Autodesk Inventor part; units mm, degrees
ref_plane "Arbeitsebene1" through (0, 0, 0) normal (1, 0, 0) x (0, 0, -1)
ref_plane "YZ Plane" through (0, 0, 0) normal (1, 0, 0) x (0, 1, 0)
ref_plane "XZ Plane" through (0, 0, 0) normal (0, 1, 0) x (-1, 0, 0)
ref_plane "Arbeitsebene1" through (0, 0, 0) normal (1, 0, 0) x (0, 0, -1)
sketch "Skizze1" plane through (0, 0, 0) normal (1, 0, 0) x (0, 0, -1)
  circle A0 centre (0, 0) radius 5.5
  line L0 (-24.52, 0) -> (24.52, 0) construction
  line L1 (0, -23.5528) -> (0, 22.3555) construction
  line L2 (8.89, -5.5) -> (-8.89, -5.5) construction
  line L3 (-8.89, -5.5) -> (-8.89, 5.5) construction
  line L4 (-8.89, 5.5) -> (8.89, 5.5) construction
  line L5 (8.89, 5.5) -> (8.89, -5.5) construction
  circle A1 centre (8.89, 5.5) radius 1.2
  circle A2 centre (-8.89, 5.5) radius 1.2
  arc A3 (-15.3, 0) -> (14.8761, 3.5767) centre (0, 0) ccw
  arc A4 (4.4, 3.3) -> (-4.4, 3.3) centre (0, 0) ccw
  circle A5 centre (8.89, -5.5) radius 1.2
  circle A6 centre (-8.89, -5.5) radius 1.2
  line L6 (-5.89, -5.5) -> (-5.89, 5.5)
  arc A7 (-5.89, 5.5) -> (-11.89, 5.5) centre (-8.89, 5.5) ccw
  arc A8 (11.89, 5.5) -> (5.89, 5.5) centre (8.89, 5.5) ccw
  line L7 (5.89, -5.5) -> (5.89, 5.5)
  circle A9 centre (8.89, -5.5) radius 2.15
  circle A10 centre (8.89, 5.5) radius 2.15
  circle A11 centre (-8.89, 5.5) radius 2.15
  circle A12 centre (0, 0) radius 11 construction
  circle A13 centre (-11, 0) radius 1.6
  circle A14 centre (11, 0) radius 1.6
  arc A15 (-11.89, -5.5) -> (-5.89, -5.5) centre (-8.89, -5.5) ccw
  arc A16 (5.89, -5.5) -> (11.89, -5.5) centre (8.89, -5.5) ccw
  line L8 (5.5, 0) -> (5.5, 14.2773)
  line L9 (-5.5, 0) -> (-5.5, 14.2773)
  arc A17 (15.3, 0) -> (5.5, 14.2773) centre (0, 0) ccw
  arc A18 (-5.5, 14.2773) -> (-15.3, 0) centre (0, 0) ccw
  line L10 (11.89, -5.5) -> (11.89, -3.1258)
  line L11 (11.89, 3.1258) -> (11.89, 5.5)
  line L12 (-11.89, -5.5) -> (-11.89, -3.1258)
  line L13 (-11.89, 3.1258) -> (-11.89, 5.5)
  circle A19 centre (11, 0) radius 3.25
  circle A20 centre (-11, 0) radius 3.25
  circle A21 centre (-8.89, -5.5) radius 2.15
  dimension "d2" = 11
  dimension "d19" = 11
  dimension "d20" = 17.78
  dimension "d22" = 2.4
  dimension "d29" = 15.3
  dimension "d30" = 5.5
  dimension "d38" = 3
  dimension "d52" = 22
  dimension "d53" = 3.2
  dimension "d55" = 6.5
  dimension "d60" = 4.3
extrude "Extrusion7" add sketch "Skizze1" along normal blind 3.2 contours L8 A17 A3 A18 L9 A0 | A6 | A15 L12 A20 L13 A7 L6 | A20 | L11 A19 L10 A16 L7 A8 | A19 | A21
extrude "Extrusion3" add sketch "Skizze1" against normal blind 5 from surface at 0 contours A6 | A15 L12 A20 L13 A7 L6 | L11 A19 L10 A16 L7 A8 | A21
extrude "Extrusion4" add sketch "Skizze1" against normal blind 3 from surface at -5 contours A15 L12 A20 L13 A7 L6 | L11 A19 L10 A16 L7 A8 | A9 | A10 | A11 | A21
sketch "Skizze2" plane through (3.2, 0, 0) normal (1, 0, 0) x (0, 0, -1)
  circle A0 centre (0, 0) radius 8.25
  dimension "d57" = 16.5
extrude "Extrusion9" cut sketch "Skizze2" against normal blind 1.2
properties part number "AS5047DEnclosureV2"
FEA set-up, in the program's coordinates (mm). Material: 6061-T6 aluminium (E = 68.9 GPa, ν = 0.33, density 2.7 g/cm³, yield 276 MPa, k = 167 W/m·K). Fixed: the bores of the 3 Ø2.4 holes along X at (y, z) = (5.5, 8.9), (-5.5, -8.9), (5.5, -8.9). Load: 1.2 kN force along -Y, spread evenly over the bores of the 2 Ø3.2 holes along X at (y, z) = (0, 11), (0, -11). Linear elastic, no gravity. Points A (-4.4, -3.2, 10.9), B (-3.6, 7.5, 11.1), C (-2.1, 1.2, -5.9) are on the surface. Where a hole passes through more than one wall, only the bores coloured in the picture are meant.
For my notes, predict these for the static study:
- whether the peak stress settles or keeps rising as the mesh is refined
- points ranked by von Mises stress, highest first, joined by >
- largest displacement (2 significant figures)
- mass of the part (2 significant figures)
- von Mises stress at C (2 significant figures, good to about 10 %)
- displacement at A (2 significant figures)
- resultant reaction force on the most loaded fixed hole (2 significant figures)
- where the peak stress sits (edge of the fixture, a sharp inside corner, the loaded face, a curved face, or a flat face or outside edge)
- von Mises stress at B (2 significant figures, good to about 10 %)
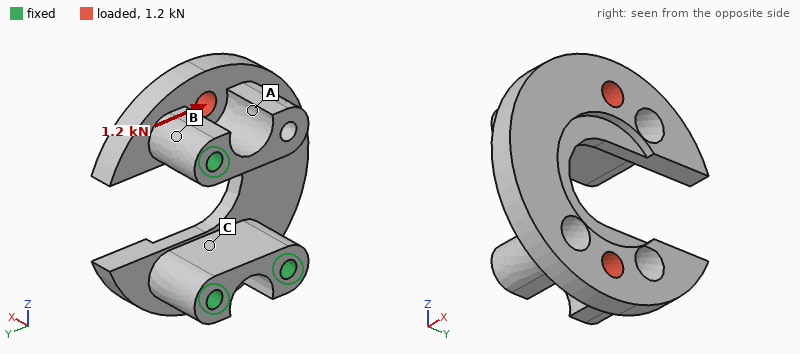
keeps rising
B > C > A
83 µm
6.1 g
38 MPa
43 µm
590 N
edge of the fixture
100 MPa
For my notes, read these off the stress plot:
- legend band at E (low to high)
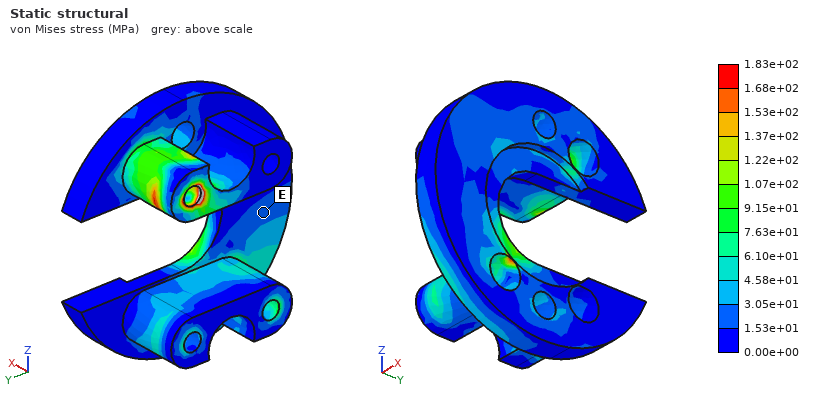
1.53e+01 to 3.05e+01 MPa
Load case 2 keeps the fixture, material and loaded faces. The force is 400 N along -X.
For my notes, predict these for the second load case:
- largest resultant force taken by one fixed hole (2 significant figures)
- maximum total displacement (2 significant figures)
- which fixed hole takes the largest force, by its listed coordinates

190 N
23 µm
(5.5, 8.9)
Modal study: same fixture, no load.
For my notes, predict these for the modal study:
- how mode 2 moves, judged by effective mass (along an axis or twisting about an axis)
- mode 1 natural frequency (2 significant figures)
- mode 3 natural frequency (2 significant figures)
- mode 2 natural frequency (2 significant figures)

along Z
8200 Hz
17 kHz
14 kHz
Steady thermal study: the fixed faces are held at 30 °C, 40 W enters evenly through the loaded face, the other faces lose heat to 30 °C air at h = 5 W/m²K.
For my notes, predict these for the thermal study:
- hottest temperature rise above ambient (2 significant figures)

45 K
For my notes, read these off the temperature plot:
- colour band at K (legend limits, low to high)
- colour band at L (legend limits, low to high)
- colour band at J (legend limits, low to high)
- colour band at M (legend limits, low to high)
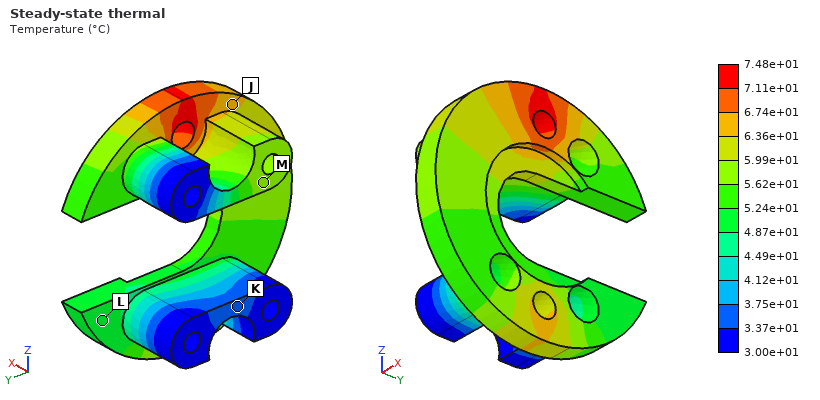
3.37e+01 to 3.75e+01 °C
4.87e+01 to 5.24e+01 °C
6.36e+01 to 6.74e+01 °C
5.62e+01 to 5.99e+01 °C
